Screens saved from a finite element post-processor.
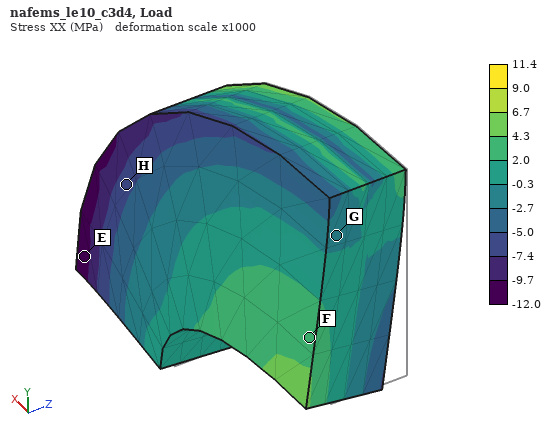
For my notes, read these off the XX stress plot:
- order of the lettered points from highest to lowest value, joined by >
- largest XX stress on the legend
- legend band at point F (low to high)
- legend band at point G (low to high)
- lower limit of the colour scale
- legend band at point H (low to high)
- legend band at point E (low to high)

F > G > H > E
11.4 MPa
2.0 to 4.3 MPa
-2.7 to -0.3 MPa
-12.0 MPa
-7.4 to -5.0 MPa
-12.0 to -9.7 MPa
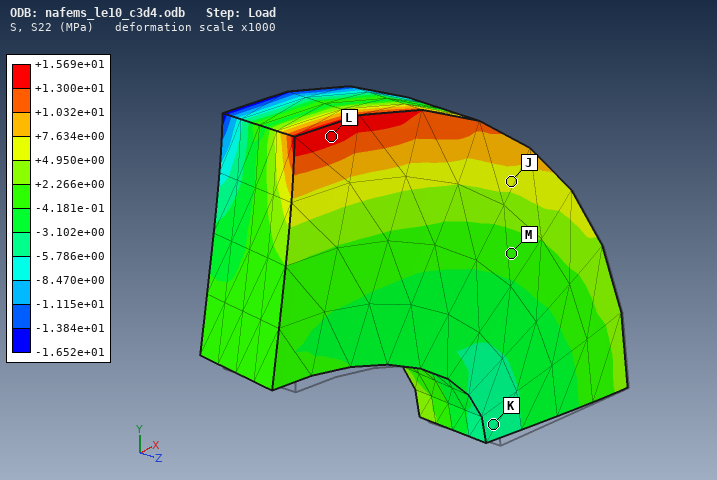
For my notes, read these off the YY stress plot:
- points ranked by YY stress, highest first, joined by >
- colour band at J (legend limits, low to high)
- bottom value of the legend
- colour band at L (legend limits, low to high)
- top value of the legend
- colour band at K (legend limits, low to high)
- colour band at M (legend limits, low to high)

L > J > M > K
+4.950e+00 to +7.634e+00 MPa
-1.652e+01 MPa
+1.300e+01 to +1.569e+01 MPa
+1.569e+01 MPa
-5.786e+00 to -3.102e+00 MPa
-4.181e-01 to +2.266e+00 MPa
